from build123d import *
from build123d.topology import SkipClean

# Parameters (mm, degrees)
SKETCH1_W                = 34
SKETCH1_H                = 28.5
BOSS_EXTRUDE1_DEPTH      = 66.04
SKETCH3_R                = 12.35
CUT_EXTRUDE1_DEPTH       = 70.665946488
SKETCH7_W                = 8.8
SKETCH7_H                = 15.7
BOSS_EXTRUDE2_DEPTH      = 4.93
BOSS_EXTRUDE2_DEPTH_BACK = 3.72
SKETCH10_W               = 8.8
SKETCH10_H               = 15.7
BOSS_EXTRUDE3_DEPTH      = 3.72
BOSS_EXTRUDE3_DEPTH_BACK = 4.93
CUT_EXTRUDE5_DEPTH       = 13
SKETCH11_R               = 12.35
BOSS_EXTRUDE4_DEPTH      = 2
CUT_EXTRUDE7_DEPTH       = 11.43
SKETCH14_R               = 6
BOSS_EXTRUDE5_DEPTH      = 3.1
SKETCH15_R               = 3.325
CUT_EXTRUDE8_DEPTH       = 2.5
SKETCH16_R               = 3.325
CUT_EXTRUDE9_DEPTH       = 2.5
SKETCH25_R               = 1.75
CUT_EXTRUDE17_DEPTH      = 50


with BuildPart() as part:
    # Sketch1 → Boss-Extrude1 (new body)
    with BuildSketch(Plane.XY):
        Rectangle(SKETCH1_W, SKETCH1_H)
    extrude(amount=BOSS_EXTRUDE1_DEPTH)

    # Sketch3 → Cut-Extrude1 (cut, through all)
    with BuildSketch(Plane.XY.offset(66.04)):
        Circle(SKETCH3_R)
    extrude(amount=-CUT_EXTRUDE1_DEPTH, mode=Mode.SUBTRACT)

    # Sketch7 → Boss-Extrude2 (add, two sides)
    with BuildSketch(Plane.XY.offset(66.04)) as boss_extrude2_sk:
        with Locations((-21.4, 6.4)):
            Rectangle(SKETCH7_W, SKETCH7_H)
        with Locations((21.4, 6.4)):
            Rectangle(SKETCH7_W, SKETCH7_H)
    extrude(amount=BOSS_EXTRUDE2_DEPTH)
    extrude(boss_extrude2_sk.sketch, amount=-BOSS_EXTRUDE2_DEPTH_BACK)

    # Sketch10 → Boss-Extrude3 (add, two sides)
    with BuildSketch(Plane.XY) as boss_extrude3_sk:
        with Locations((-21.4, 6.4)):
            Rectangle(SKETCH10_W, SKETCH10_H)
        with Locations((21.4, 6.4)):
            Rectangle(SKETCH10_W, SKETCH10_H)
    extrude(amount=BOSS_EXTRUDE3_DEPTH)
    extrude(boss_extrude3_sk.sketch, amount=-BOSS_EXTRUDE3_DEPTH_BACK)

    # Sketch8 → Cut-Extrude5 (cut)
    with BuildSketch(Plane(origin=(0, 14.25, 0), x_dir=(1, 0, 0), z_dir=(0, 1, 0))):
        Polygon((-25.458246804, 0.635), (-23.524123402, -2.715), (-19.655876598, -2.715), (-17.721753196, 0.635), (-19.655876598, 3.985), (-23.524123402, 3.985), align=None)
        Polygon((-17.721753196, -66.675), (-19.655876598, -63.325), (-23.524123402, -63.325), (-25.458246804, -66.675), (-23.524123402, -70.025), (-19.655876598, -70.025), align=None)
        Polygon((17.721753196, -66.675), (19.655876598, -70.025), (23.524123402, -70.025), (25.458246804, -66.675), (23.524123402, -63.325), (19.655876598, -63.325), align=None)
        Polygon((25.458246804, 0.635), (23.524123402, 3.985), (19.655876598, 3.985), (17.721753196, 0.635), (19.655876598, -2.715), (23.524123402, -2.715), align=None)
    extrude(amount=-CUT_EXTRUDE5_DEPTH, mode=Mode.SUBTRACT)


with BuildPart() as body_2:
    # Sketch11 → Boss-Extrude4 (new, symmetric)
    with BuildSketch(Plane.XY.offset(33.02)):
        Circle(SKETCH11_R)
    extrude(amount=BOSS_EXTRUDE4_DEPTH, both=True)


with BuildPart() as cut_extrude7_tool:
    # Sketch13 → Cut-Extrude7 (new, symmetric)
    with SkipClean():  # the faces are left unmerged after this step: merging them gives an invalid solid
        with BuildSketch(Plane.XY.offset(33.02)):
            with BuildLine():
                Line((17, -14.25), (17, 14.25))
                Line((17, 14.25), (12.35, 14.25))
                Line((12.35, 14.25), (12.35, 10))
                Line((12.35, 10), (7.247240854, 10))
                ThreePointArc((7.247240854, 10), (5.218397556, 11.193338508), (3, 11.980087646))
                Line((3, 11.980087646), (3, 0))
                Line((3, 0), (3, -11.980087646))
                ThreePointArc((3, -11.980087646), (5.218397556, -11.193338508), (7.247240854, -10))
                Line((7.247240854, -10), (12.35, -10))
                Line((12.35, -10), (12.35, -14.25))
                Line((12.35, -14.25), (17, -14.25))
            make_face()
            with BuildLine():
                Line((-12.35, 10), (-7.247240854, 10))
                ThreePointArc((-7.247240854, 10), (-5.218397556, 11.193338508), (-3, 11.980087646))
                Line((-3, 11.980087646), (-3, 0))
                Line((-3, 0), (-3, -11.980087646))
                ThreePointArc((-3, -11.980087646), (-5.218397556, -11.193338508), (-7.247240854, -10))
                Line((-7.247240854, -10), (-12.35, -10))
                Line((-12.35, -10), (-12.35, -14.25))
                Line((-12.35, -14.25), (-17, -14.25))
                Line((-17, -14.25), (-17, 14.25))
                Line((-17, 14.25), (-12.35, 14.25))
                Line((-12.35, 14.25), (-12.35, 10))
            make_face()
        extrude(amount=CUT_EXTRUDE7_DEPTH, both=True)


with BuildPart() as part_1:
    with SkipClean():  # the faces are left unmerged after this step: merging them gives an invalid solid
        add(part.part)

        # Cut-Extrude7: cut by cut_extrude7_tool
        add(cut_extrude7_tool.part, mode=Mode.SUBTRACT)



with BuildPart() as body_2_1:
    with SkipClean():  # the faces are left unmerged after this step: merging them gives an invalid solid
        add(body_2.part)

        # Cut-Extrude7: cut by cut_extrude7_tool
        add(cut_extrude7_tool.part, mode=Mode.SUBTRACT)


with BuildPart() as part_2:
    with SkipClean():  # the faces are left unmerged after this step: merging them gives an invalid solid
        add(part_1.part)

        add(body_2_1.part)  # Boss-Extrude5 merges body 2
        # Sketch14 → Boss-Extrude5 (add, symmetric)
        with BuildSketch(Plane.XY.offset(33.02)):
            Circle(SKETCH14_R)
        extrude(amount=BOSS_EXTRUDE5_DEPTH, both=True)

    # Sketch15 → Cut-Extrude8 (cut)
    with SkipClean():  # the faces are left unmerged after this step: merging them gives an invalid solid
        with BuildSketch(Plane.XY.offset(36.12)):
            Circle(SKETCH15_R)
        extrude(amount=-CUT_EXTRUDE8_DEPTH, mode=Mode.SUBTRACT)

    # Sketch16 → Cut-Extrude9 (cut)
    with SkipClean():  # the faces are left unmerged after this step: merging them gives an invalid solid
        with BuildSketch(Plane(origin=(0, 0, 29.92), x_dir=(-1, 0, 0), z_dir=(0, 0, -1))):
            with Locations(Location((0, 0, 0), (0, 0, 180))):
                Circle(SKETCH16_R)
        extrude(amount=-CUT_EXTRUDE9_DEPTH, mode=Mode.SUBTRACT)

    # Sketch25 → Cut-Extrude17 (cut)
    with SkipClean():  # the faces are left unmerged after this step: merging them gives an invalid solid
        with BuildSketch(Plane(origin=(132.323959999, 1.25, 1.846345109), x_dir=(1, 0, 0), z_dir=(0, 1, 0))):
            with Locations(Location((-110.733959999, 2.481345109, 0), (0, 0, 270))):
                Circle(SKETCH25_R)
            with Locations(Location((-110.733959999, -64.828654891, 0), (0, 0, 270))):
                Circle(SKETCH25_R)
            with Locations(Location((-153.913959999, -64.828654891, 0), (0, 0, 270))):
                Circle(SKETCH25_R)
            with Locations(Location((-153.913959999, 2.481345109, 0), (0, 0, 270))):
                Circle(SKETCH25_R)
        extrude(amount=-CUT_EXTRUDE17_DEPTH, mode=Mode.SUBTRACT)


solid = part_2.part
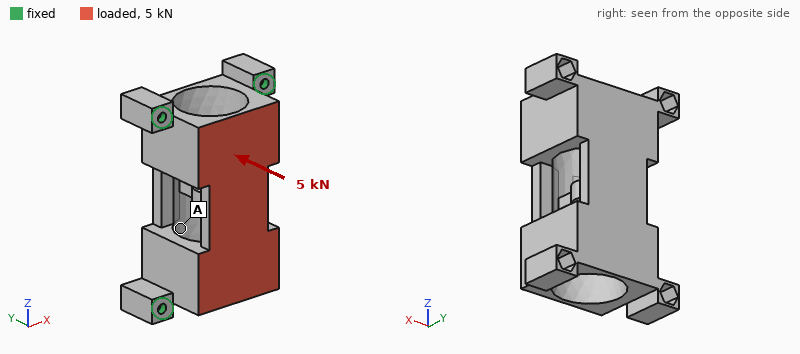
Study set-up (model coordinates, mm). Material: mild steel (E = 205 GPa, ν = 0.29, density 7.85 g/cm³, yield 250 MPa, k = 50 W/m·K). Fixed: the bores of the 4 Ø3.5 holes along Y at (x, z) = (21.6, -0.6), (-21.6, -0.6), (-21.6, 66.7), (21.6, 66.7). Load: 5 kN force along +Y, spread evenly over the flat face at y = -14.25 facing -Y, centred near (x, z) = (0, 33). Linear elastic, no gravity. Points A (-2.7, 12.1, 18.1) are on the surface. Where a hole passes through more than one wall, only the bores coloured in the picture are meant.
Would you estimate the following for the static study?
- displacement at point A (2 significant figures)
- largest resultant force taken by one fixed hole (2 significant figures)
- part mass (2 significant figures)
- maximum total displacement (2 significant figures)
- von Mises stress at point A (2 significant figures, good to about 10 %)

6.1 µm
1.3 kN
220 g
14 µm
17 MPa
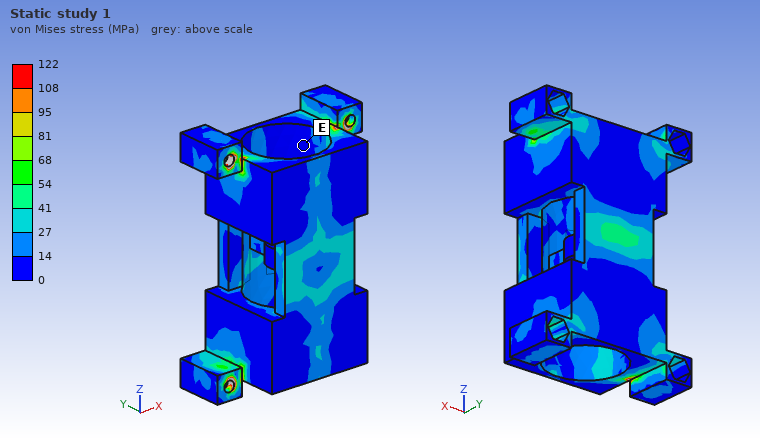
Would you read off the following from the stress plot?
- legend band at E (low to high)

0 to 14 MPa
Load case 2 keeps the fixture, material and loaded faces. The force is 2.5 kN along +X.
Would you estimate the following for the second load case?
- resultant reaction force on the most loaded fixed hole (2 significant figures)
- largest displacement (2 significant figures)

850 N
11 µm
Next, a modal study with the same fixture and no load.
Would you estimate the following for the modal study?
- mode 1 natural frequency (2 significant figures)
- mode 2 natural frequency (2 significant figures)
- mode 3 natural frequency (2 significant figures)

7800 Hz
8600 Hz
8800 Hz
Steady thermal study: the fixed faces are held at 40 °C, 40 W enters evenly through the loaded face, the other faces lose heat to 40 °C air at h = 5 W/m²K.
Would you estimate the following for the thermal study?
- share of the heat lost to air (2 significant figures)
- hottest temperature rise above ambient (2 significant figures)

8.2 %
78 K
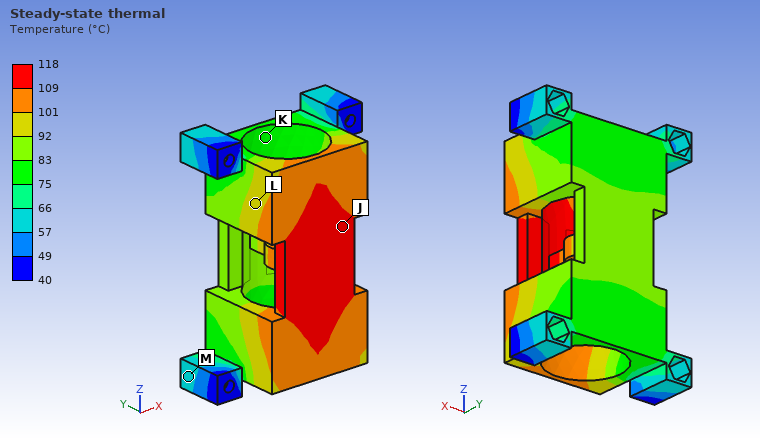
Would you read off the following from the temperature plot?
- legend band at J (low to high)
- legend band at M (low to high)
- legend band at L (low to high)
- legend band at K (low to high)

109 to 118 °C
57 to 66 °C
92 to 101 °C
75 to 83 °C
